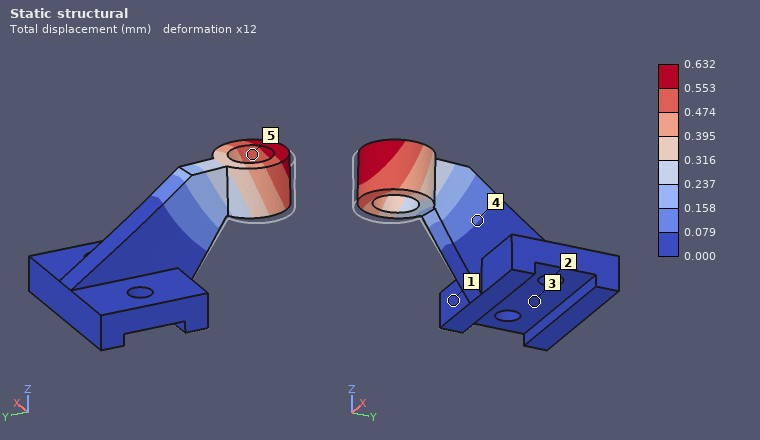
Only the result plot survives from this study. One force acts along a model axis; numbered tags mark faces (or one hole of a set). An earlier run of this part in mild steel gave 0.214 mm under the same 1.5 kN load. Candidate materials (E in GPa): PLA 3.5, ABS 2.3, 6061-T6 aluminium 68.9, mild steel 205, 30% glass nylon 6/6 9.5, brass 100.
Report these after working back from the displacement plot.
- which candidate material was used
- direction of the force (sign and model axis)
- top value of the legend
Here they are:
6061-T6 aluminium
+X
0.632 mm
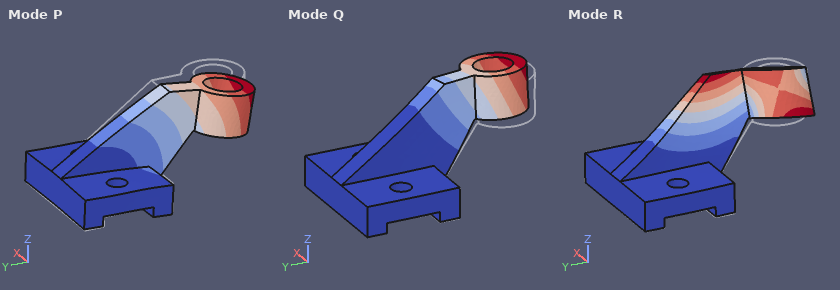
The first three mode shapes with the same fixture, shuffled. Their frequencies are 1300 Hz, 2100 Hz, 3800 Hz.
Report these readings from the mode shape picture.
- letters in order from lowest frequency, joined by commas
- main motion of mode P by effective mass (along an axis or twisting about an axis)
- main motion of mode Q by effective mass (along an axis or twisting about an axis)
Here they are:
Q, P, R
along Z
along X
